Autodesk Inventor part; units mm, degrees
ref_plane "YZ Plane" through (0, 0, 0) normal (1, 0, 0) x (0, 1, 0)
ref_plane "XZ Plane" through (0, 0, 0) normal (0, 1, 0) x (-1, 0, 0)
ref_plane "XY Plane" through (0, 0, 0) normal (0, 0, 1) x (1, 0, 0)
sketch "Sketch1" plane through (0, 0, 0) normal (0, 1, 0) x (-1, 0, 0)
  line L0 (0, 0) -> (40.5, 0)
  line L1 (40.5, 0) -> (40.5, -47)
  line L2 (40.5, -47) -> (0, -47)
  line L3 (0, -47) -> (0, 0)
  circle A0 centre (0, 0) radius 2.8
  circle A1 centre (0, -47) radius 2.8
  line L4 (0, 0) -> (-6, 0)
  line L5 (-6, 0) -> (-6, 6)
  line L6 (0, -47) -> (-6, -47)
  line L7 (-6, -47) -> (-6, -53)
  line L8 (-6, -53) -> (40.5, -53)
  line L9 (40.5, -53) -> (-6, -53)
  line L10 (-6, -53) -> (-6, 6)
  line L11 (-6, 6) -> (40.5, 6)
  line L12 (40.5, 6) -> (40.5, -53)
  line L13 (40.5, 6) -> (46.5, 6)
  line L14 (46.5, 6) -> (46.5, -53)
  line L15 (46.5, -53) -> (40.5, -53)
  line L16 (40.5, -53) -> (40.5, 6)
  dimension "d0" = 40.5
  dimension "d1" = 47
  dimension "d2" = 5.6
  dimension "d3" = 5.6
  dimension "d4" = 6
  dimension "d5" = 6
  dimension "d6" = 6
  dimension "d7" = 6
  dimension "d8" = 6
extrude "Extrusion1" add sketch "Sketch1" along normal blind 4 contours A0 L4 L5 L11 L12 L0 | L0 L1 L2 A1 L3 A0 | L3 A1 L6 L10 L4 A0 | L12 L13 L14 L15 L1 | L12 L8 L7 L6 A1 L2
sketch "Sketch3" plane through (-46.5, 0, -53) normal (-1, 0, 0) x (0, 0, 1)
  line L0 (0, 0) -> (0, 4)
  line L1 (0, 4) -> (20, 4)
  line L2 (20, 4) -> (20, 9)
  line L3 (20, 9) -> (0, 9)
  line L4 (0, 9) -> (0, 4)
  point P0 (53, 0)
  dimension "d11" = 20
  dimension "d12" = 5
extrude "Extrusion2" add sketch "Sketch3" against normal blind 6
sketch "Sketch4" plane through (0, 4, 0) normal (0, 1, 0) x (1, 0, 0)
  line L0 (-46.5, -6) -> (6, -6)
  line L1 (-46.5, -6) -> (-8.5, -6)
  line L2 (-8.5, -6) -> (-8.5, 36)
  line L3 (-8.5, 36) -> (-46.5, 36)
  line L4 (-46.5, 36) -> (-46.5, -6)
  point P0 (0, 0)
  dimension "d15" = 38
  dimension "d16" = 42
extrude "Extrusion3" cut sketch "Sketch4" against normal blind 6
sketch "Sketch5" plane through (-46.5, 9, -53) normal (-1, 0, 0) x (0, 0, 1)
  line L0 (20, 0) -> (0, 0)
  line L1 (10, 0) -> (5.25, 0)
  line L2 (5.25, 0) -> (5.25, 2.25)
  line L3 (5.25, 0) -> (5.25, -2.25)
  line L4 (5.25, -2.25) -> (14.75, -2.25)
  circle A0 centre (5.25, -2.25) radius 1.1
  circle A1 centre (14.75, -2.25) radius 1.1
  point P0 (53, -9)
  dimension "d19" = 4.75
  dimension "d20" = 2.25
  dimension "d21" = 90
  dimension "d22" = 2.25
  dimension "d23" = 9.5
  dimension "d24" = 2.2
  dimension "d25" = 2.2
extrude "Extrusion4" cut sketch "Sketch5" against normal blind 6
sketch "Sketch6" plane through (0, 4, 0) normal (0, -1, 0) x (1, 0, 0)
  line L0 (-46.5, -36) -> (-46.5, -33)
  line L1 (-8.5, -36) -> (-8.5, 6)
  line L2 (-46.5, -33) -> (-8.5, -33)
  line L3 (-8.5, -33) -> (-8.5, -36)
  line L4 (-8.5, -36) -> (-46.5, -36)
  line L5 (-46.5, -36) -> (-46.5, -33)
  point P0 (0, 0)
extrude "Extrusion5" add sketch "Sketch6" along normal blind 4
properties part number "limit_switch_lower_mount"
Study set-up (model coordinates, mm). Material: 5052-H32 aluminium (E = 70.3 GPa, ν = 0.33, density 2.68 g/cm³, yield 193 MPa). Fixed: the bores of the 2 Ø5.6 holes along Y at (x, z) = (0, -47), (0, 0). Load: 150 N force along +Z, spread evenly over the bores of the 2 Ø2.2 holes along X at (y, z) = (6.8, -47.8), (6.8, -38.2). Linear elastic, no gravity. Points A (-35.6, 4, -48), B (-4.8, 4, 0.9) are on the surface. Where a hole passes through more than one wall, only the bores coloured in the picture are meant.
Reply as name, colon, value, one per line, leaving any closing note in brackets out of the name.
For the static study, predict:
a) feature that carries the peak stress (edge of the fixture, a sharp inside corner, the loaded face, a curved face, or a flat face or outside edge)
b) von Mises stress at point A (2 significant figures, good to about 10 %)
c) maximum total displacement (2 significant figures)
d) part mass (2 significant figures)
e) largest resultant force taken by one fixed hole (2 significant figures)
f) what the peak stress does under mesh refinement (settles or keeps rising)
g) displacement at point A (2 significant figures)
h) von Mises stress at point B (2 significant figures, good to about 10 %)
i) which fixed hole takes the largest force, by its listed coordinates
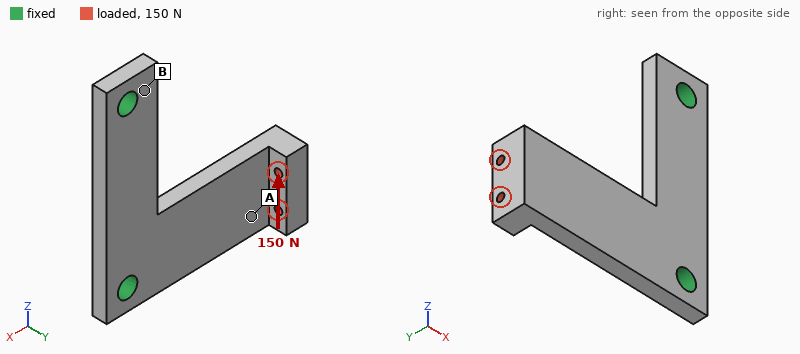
feature that carries the peak stress: edge of the fixture
von Mises stress at point A: 15 MPa
maximum total displacement: 61 µm
part mass: 18 g
largest resultant force taken by one fixed hole: 140 N
what the peak stress does under mesh refinement: keeps rising
displacement at point A: 30 µm
von Mises stress at point B: 4.1 MPa
which fixed hole takes the largest force, by its listed coordinates: (0, 0)
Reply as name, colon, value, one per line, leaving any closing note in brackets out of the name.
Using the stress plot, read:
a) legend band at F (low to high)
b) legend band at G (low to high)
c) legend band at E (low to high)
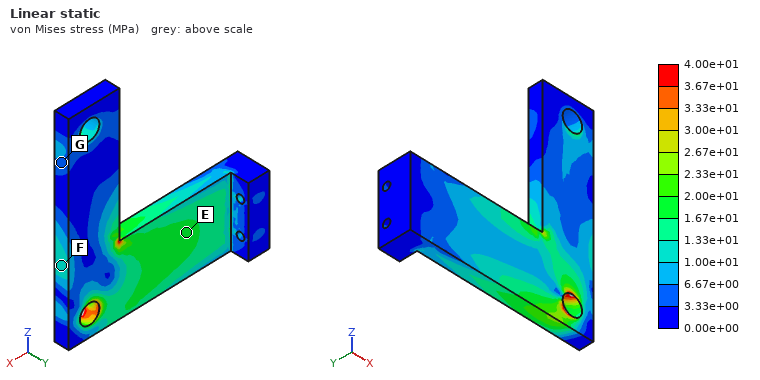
legend band at F: 1.00e+01 to 1.33e+01 MPa
legend band at G: 3.33e+00 to 6.67e+00 MPa
legend band at E: 1.67e+01 to 2.00e+01 MPa
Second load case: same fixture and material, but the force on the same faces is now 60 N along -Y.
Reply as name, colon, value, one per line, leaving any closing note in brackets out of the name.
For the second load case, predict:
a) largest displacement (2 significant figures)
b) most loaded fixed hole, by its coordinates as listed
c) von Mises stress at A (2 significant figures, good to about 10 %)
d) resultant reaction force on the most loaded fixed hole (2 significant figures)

largest displacement: 0.23 mm
most loaded fixed hole, by its coordinates as listed: (0, -47)
von Mises stress at A: 9.1 MPa
resultant reaction force on the most loaded fixed hole: 64 N
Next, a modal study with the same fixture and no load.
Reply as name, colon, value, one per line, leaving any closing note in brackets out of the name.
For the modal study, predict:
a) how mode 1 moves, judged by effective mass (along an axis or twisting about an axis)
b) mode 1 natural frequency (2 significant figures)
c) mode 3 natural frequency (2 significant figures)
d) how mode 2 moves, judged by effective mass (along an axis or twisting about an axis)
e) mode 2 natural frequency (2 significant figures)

how mode 1 moves, judged by effective mass: along Y
mode 1 natural frequency: 1300 Hz
mode 3 natural frequency: 5800 Hz
how mode 2 moves, judged by effective mass: along Z
mode 2 natural frequency: 4700 Hz
